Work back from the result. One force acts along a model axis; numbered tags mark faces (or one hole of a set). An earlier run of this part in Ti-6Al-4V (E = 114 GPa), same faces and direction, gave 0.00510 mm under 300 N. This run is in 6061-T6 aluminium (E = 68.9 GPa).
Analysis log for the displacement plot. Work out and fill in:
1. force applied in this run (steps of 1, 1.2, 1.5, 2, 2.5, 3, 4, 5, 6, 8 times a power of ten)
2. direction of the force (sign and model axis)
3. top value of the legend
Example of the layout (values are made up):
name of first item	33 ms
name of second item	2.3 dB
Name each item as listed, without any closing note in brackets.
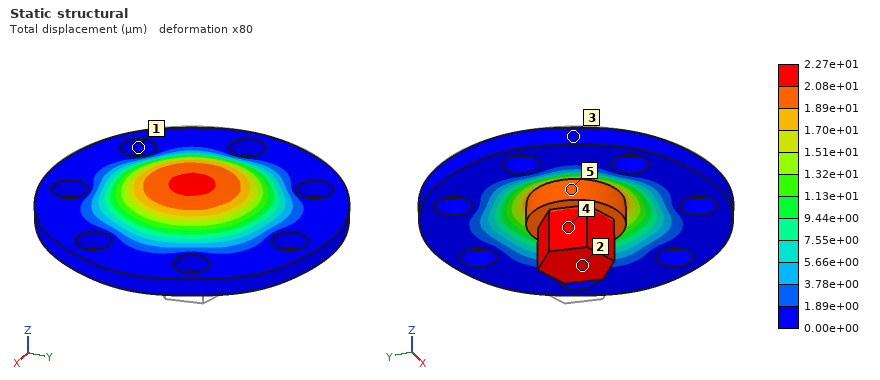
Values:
force applied in this run	800 N
direction of the force	+Z
top value of the legend	2.27e+01 µm
